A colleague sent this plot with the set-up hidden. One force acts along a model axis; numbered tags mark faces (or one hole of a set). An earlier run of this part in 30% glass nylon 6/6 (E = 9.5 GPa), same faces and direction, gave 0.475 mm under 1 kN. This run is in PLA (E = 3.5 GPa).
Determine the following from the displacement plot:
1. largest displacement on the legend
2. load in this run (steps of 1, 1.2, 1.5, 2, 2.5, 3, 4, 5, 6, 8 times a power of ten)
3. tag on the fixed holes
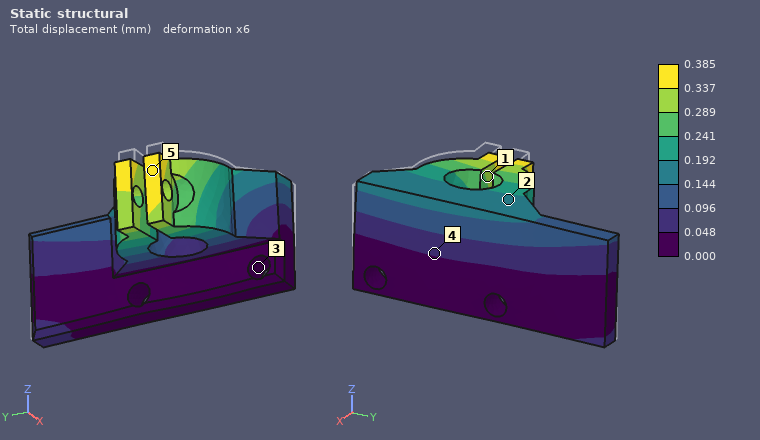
0.385 mm
300 N
3
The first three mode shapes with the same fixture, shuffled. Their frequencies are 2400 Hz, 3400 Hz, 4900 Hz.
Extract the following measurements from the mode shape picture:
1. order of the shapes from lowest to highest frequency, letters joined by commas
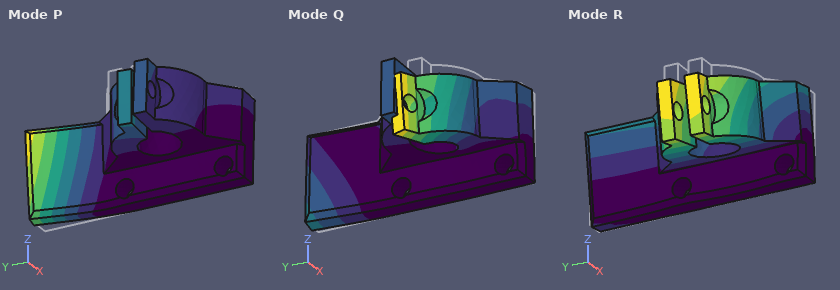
R, P, Q
